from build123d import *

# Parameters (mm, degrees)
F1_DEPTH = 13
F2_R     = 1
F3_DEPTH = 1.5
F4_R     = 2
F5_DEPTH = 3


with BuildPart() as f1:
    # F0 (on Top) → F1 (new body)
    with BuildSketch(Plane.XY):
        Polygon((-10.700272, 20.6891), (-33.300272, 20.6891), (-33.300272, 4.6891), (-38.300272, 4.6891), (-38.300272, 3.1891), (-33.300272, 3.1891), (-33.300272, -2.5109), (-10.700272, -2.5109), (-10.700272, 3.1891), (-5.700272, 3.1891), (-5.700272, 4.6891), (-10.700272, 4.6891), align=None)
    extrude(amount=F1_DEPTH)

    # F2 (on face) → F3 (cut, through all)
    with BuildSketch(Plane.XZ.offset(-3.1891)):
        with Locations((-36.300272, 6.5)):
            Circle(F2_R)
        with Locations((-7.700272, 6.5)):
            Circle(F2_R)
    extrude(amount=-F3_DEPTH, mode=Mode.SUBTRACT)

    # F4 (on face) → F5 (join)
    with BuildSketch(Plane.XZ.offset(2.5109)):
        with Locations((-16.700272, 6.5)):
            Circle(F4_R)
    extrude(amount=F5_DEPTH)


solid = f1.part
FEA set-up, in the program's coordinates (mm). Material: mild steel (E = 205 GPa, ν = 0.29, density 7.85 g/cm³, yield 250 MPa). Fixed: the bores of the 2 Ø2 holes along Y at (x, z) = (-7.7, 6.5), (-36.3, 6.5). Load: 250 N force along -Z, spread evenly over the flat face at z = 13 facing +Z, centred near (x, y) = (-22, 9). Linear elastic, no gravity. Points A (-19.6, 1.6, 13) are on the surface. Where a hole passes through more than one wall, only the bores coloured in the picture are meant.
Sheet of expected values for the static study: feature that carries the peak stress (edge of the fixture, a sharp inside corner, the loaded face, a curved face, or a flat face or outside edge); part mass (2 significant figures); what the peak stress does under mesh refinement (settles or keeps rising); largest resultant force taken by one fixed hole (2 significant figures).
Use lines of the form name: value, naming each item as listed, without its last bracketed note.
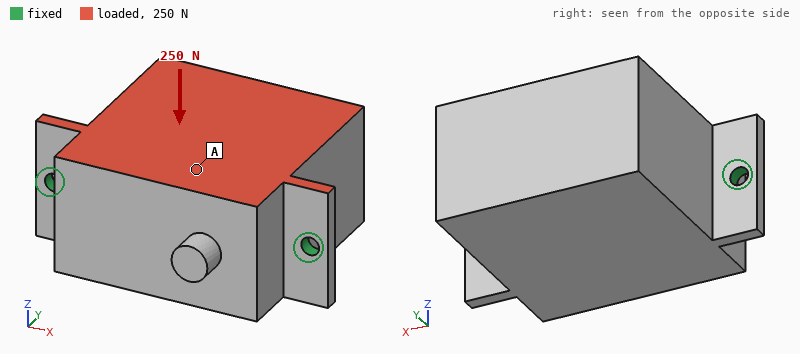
feature that carries the peak stress: edge of the fixture
part mass: 55 g
what the peak stress does under mesh refinement: keeps rising
largest resultant force taken by one fixed hole: 130 N
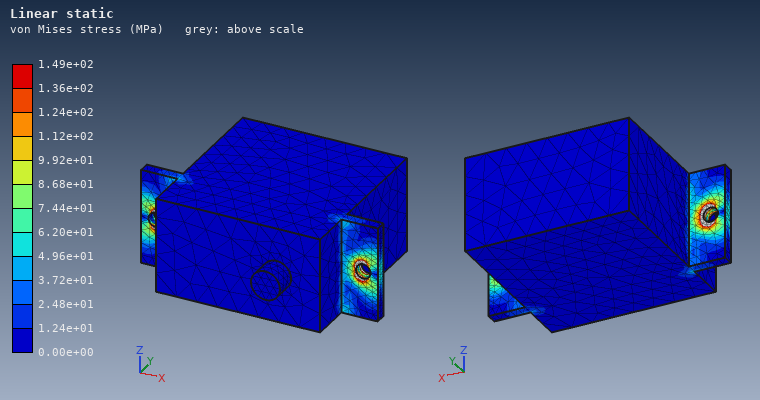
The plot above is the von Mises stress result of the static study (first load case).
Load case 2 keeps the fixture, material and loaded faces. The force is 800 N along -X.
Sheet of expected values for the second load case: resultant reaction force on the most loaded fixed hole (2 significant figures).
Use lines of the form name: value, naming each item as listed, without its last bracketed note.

resultant reaction force on the most loaded fixed hole: 470 N
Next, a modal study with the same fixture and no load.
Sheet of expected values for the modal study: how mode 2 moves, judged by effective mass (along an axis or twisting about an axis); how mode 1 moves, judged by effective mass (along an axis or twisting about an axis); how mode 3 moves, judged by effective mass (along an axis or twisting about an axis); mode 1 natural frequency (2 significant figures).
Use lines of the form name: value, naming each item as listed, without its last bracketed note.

how mode 2 moves, judged by effective mass: along Y
how mode 1 moves, judged by effective mass: along Z
how mode 3 moves, judged by effective mass: along X
mode 1 natural frequency: 2100 Hz
